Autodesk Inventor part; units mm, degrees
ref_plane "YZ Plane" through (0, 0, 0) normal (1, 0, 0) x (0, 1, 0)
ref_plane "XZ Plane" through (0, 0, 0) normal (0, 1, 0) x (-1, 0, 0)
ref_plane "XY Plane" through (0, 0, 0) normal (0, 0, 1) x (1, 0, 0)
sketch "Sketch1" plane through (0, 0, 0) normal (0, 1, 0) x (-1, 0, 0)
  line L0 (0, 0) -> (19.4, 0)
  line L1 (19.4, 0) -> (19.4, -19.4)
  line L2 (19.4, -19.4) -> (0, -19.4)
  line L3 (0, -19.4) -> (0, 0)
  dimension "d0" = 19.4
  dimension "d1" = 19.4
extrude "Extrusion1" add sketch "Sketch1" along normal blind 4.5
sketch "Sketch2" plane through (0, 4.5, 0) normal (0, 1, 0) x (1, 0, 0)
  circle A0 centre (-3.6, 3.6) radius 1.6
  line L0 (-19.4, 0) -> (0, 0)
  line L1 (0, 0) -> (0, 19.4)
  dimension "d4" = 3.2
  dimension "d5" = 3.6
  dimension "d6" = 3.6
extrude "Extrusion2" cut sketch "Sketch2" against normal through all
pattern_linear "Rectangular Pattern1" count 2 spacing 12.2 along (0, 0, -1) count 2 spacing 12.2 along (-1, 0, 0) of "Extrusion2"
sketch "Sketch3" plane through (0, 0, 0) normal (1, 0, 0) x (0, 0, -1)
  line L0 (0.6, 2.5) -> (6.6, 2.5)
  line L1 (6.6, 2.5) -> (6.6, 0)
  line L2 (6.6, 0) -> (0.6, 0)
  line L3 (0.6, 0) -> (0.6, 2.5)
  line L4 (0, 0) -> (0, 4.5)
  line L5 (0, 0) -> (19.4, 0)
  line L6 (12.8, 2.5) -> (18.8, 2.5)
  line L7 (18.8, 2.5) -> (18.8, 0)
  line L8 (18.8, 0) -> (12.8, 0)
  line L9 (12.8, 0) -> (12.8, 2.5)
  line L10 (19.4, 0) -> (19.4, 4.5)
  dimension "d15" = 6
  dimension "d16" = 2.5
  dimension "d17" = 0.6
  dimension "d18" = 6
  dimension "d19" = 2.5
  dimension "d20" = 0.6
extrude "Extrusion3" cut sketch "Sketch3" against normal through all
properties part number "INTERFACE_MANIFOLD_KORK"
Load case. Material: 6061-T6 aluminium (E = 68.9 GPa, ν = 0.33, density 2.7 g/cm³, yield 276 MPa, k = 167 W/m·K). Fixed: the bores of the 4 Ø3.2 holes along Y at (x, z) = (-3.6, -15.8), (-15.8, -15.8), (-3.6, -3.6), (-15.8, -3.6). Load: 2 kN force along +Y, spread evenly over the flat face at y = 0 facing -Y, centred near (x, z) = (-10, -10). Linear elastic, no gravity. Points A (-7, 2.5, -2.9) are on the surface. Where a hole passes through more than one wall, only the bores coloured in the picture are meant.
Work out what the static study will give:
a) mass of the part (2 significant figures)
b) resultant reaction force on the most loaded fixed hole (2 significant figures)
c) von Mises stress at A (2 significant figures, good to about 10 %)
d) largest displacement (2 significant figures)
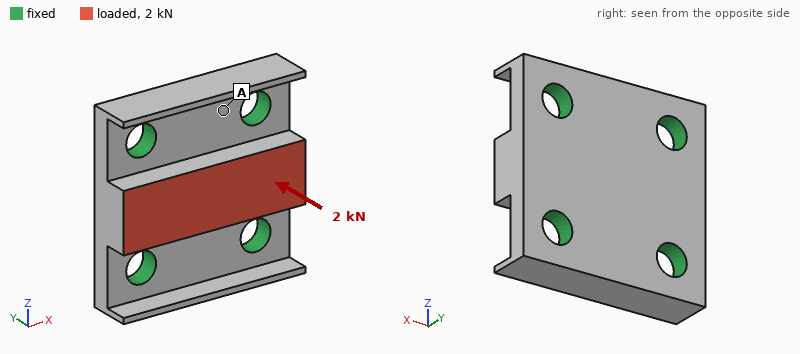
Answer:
2.8 g
540 N
22 MPa
9.4 µm
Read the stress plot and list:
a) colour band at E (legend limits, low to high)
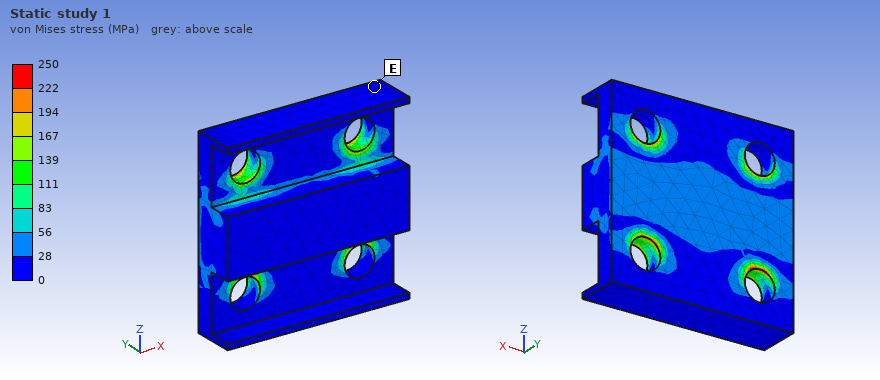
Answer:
0 to 28 MPa
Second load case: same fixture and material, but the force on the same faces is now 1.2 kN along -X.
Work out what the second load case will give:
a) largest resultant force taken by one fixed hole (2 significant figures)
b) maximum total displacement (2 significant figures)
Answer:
360 N
9.0 µm
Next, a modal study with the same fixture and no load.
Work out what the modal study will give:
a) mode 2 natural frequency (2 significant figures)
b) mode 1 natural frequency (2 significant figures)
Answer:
58 kHz
58 kHz
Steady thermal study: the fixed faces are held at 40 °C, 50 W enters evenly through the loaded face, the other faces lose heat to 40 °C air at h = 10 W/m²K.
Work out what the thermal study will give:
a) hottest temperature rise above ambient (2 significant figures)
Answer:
22 K
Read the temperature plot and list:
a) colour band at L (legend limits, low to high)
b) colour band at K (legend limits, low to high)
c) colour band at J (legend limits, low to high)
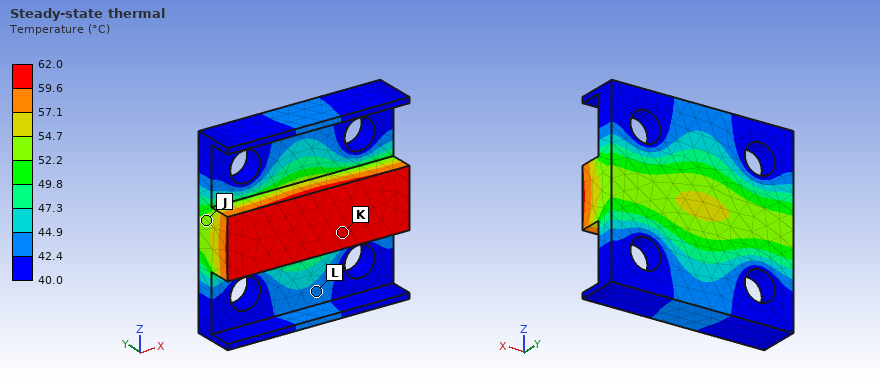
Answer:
42.4 to 44.9 °C
59.6 to 62.0 °C
52.2 to 54.7 °C
